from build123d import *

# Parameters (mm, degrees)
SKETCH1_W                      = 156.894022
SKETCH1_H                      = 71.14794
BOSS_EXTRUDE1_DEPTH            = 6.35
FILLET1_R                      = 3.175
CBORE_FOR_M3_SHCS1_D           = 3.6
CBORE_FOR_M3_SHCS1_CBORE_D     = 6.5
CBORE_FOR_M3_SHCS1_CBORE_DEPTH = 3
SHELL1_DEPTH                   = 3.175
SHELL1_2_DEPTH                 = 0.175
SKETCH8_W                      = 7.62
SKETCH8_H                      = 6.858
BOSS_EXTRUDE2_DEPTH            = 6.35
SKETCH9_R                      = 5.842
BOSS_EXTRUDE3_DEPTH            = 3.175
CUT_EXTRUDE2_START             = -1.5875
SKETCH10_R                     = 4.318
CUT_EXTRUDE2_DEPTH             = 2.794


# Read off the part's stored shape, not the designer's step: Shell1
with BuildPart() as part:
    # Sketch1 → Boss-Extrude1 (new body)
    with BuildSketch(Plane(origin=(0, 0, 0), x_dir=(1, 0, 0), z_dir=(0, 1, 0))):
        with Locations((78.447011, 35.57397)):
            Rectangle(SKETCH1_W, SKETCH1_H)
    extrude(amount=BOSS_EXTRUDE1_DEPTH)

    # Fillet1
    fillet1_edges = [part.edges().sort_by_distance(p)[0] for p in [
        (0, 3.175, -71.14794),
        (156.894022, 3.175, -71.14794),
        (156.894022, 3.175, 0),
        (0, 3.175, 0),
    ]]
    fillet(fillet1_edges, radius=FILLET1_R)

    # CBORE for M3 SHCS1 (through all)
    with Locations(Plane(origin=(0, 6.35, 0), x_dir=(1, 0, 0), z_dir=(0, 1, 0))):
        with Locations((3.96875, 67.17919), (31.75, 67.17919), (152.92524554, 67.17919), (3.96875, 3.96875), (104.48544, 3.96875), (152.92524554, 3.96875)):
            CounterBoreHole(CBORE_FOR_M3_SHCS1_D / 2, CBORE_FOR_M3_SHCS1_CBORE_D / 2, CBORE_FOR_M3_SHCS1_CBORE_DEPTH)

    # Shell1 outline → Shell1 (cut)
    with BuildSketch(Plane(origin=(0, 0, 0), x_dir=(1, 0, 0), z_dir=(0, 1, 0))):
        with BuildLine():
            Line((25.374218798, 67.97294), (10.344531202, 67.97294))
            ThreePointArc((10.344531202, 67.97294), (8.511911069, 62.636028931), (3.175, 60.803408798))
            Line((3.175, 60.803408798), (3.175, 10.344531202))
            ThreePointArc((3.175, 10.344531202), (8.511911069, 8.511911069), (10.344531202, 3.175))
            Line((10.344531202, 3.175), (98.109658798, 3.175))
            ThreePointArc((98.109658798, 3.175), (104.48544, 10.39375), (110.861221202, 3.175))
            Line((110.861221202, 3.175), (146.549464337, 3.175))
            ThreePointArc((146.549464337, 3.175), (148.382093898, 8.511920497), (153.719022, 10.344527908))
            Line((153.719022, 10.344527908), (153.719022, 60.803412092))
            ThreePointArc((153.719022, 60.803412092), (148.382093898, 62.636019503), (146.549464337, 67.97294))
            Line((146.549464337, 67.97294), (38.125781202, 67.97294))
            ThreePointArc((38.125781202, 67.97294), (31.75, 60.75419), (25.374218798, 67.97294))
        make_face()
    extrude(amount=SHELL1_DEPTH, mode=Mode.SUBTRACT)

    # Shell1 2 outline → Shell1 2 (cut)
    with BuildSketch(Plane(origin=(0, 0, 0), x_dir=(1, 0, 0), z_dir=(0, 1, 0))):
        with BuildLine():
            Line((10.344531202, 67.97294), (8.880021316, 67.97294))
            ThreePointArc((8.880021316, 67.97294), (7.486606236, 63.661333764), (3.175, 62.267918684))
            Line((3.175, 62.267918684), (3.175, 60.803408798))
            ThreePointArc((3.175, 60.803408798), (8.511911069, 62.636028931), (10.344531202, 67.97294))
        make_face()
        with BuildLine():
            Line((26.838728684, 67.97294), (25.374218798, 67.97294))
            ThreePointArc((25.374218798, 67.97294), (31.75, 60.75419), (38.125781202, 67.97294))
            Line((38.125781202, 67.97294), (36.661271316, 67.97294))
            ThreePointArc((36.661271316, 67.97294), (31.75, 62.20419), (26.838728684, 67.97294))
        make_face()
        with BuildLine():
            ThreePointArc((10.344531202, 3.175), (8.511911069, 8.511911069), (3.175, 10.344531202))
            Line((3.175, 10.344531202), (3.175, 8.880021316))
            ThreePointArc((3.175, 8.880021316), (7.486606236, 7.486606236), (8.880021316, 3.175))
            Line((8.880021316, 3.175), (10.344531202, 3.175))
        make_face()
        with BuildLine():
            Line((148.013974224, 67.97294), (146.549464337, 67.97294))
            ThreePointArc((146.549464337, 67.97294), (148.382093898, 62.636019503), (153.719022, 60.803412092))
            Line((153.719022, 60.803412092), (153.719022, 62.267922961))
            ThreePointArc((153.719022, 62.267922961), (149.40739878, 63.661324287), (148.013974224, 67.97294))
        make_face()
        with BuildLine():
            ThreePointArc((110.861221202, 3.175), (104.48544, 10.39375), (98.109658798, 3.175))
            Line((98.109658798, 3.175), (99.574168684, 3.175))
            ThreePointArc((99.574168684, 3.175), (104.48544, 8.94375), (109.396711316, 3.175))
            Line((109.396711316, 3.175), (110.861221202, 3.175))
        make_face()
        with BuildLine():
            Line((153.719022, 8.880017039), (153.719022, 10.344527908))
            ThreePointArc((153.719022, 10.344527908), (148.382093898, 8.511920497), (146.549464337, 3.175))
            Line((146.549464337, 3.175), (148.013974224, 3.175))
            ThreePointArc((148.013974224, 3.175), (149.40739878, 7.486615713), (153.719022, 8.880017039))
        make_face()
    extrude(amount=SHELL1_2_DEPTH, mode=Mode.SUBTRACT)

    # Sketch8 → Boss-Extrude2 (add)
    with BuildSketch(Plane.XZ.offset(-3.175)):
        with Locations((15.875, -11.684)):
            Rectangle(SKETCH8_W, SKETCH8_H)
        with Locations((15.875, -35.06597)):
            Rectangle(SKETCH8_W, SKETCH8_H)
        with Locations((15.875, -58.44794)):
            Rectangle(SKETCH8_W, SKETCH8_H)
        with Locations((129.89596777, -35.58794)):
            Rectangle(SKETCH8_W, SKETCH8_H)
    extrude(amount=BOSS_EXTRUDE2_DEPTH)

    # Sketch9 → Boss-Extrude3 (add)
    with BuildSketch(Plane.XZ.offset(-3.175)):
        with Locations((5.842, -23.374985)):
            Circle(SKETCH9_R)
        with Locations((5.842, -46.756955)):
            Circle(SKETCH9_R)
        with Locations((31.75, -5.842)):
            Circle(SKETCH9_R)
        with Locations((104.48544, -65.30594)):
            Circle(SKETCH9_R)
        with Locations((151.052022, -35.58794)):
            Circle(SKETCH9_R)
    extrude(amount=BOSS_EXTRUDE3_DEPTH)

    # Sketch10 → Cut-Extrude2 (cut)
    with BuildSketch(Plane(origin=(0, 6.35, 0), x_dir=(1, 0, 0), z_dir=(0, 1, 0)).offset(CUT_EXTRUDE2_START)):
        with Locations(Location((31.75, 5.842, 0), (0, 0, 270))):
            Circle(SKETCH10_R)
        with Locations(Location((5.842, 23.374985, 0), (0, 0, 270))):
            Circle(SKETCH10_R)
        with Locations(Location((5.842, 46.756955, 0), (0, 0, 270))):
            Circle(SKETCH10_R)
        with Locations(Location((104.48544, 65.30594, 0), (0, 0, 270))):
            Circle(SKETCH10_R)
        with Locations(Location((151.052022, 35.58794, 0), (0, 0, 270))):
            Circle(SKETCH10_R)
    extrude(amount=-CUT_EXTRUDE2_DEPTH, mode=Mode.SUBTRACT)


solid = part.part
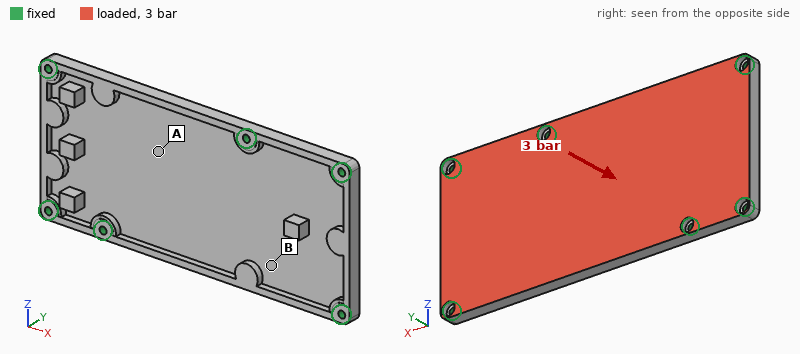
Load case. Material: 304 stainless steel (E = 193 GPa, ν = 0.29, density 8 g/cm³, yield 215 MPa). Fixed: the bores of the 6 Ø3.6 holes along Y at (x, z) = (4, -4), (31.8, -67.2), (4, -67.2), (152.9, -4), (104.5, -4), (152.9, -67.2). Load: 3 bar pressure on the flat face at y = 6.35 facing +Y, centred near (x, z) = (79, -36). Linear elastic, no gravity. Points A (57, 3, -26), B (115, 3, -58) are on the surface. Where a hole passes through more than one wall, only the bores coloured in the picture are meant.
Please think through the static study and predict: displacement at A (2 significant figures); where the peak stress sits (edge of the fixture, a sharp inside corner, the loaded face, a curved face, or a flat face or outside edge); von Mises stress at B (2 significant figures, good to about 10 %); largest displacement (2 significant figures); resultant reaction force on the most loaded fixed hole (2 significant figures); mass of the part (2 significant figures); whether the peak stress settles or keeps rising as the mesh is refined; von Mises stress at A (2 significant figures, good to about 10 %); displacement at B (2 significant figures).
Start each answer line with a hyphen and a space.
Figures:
- 0.10 mm
- edge of the fixture
- 22 MPa
- 0.14 mm
- 1.9 kN
- 340 g
- keeps rising
- 42 MPa
- 0.10 mm
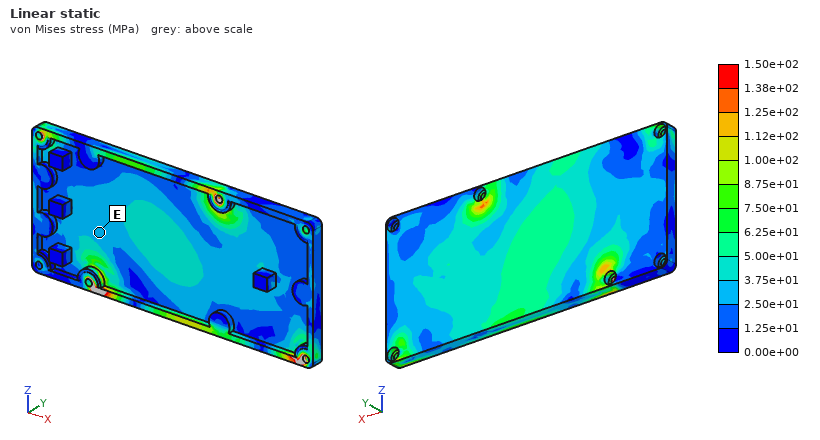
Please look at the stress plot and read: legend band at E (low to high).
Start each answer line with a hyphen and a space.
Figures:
- 2.50e+01 to 3.75e+01 MPa
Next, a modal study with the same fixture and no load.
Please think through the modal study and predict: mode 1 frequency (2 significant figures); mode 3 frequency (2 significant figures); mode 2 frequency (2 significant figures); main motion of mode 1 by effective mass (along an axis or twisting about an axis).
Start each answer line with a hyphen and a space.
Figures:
- 1700 Hz
- 3600 Hz
- 2300 Hz
- along Y
